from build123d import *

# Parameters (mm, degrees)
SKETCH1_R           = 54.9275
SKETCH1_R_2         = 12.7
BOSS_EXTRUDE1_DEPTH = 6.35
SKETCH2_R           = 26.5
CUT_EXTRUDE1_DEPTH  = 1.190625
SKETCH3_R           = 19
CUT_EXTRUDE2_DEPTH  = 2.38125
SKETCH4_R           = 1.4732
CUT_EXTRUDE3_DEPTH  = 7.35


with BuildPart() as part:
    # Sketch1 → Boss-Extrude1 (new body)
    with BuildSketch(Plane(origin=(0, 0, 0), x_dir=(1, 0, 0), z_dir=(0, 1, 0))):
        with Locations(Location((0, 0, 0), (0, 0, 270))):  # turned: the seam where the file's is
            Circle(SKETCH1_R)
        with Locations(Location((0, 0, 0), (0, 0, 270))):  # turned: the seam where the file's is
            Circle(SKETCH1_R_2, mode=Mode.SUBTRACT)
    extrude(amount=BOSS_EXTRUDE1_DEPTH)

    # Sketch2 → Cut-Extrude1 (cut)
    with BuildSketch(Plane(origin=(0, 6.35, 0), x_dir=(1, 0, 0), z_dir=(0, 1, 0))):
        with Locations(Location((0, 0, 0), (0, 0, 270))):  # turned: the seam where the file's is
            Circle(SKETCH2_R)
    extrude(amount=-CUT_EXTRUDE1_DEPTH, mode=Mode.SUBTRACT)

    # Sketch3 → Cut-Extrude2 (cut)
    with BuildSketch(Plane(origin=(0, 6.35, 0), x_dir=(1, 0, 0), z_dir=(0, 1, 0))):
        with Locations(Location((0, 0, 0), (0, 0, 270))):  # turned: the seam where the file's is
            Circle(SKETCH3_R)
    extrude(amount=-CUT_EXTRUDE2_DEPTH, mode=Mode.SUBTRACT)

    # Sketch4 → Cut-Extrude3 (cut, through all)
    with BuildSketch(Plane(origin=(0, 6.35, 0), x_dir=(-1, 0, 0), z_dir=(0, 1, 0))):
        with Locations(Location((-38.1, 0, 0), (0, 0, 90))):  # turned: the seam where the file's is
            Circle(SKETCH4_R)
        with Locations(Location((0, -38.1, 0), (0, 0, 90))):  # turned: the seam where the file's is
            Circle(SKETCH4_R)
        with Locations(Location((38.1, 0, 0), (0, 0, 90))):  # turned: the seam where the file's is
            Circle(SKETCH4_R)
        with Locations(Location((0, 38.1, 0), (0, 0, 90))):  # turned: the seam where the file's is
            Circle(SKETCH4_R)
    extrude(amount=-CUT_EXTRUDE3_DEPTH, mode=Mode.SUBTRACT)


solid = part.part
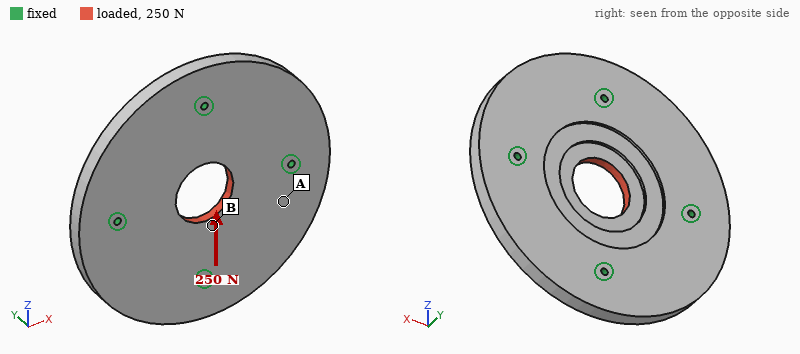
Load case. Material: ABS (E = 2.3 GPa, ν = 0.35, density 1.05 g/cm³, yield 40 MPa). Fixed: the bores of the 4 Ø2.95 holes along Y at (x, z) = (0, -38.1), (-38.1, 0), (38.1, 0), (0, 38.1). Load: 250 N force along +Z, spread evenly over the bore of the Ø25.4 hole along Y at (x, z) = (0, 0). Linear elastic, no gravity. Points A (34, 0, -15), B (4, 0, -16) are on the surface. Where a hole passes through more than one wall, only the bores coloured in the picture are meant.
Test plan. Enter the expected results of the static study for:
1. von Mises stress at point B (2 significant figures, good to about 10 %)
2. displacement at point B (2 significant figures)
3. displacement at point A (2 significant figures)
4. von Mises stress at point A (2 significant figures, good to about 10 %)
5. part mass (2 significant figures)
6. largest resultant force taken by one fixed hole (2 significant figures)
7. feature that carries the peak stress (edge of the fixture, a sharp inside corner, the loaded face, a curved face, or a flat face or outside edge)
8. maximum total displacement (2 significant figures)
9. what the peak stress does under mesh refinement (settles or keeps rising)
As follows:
0.89 MPa
10 µm
3.4 µm
0.22 MPa
57 g
75 N
edge of the fixture
12 µm
keeps rising
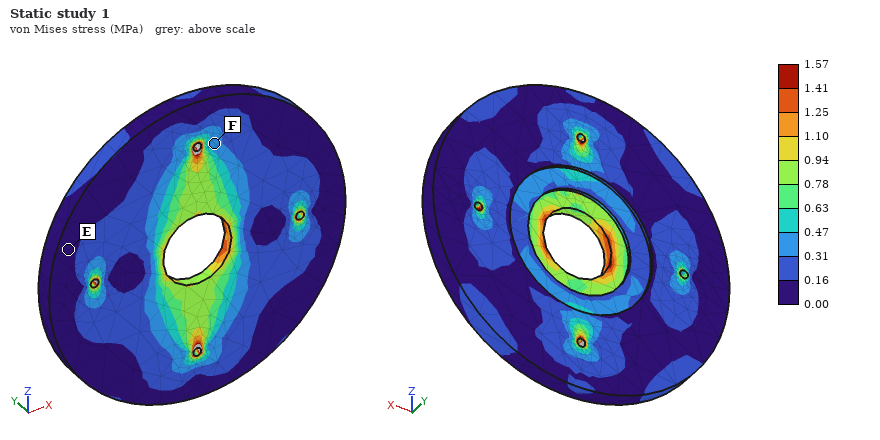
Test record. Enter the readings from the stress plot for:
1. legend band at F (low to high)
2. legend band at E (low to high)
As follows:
0.31 to 0.47 MPa
0.00 to 0.16 MPa
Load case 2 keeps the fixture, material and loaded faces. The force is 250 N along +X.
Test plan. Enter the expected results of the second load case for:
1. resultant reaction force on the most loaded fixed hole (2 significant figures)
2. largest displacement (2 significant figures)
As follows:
75 N
12 µm
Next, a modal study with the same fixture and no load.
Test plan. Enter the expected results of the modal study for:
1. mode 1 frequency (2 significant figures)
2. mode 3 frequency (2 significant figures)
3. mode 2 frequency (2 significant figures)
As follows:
1300 Hz
1600 Hz
1600 Hz
